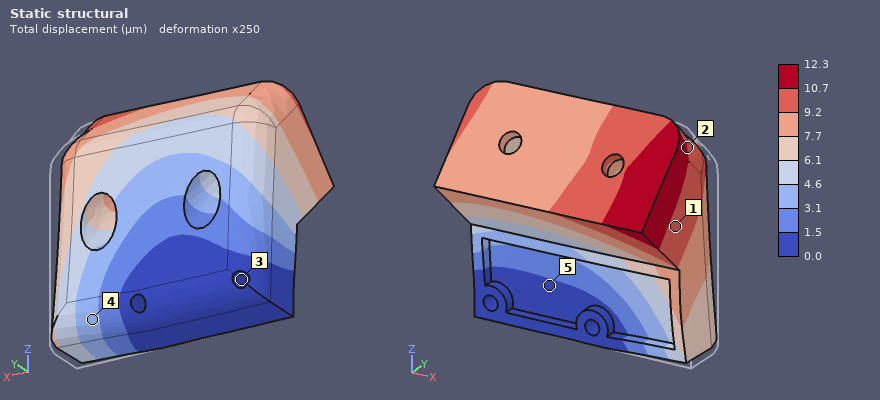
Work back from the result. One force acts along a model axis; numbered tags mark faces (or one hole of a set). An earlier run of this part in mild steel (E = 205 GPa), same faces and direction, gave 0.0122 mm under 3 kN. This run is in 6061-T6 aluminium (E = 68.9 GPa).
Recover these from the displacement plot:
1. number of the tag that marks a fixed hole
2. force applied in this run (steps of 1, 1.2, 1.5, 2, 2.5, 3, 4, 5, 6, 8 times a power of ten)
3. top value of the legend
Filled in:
3
1 kN
12.3 µm
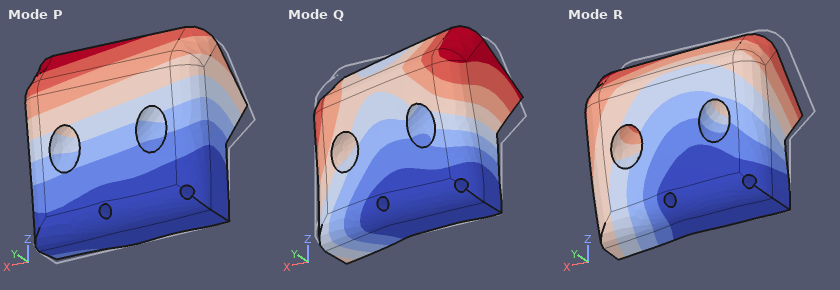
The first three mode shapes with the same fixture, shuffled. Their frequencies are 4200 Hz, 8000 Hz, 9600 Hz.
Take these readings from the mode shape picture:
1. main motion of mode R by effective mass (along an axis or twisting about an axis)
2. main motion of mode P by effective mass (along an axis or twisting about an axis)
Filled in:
along X
along Y
